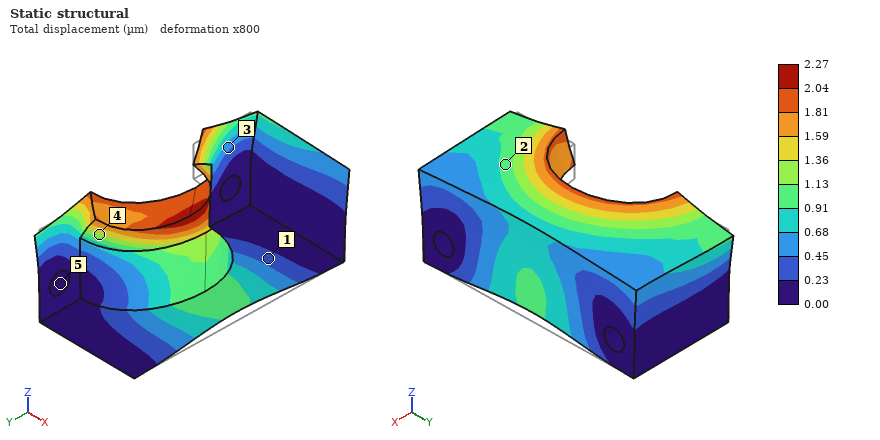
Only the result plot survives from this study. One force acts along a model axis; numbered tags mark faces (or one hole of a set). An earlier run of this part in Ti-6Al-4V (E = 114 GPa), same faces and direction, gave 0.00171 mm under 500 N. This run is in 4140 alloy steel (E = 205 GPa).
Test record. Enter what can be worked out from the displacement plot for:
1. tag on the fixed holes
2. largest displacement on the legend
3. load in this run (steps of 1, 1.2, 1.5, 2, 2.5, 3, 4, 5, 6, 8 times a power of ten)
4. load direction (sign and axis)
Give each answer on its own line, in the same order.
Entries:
5
2.27 µm
1.2 kN
+Z
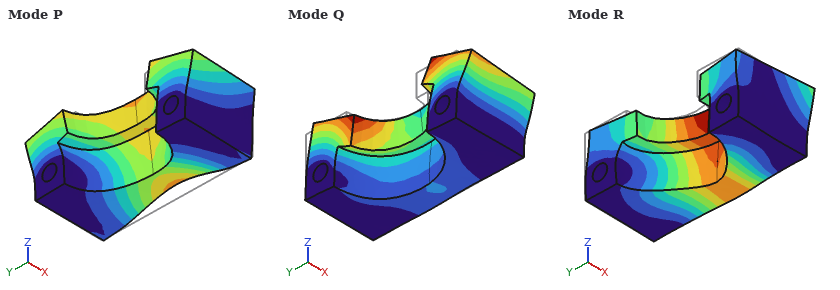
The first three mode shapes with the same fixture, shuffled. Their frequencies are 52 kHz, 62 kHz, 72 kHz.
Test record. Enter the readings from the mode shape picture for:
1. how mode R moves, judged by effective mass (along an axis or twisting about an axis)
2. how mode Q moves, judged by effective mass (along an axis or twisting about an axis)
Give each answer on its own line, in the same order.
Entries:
along X
along Y
